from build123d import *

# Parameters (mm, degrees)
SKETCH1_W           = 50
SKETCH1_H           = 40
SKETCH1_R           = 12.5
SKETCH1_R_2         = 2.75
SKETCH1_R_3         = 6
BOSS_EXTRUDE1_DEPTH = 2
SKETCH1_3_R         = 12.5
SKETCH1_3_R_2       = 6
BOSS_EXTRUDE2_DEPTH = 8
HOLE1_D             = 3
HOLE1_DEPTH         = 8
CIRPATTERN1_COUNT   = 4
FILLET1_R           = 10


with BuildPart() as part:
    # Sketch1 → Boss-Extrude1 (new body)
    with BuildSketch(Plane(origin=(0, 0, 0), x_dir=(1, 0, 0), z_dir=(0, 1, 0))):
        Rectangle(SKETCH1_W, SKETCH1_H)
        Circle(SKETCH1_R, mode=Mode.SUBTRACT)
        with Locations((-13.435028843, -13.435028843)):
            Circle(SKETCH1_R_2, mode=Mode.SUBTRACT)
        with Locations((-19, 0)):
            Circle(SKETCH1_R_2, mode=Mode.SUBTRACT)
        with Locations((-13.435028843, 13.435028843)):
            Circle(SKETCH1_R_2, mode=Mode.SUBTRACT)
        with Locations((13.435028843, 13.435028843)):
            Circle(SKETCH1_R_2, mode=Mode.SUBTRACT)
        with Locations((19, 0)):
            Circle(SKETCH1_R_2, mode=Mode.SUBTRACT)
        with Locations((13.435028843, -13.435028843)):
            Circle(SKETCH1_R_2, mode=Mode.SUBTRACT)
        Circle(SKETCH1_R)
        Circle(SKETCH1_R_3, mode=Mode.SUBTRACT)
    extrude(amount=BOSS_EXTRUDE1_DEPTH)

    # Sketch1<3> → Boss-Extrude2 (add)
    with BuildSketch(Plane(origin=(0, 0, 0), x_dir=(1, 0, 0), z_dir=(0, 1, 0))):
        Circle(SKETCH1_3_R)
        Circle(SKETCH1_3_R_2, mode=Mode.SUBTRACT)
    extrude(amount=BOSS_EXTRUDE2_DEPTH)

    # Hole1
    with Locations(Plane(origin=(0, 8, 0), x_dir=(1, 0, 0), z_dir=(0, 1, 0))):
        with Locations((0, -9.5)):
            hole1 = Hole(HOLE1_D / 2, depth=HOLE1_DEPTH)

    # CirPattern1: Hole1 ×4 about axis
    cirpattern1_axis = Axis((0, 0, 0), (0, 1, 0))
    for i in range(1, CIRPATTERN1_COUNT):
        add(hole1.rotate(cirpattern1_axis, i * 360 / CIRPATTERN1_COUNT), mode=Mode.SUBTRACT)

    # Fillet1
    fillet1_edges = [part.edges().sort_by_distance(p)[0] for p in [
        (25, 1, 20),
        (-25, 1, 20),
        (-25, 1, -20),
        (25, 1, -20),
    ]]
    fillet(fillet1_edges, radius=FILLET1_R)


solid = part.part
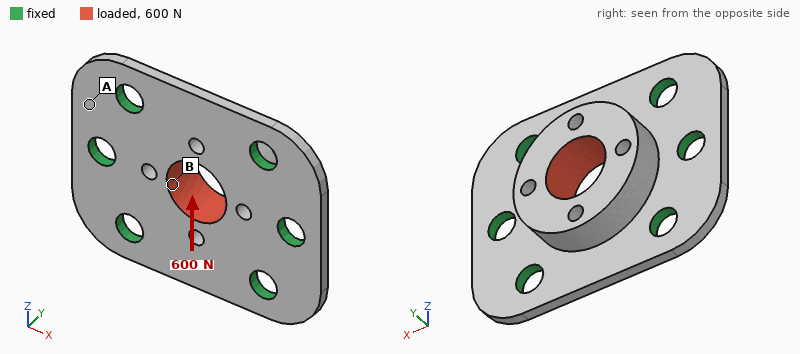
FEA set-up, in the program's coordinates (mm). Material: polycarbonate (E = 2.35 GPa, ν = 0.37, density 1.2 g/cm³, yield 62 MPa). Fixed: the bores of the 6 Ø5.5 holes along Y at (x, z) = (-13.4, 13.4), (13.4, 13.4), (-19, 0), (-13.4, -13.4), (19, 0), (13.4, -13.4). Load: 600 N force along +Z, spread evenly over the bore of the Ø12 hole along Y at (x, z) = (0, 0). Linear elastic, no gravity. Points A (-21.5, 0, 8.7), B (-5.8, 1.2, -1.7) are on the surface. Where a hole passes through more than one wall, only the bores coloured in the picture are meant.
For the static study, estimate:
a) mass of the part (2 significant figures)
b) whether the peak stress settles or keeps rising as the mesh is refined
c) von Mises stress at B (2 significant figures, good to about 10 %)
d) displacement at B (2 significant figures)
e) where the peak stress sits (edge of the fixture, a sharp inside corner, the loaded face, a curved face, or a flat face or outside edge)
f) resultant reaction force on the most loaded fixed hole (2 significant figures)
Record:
6.4 g
keeps rising
4.3 MPa
32 µm
edge of the fixture
150 N
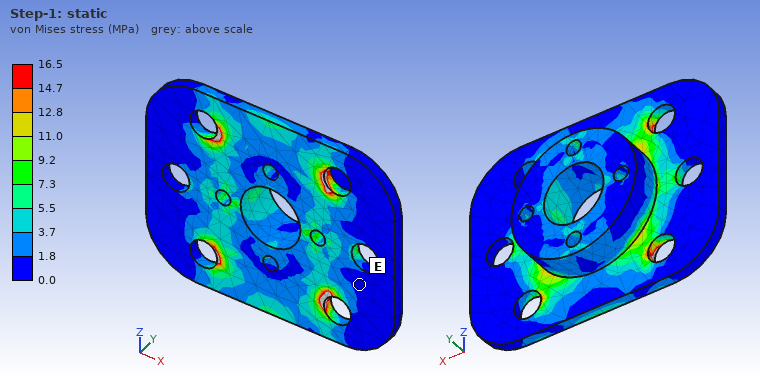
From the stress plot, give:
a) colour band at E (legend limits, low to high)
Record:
0.0 to 1.8 MPa
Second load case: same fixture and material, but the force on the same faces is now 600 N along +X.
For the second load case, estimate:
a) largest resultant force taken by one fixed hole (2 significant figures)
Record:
130 N
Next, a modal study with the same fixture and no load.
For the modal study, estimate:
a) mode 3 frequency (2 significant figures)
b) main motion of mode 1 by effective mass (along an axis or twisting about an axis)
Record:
7700 Hz
along Y
